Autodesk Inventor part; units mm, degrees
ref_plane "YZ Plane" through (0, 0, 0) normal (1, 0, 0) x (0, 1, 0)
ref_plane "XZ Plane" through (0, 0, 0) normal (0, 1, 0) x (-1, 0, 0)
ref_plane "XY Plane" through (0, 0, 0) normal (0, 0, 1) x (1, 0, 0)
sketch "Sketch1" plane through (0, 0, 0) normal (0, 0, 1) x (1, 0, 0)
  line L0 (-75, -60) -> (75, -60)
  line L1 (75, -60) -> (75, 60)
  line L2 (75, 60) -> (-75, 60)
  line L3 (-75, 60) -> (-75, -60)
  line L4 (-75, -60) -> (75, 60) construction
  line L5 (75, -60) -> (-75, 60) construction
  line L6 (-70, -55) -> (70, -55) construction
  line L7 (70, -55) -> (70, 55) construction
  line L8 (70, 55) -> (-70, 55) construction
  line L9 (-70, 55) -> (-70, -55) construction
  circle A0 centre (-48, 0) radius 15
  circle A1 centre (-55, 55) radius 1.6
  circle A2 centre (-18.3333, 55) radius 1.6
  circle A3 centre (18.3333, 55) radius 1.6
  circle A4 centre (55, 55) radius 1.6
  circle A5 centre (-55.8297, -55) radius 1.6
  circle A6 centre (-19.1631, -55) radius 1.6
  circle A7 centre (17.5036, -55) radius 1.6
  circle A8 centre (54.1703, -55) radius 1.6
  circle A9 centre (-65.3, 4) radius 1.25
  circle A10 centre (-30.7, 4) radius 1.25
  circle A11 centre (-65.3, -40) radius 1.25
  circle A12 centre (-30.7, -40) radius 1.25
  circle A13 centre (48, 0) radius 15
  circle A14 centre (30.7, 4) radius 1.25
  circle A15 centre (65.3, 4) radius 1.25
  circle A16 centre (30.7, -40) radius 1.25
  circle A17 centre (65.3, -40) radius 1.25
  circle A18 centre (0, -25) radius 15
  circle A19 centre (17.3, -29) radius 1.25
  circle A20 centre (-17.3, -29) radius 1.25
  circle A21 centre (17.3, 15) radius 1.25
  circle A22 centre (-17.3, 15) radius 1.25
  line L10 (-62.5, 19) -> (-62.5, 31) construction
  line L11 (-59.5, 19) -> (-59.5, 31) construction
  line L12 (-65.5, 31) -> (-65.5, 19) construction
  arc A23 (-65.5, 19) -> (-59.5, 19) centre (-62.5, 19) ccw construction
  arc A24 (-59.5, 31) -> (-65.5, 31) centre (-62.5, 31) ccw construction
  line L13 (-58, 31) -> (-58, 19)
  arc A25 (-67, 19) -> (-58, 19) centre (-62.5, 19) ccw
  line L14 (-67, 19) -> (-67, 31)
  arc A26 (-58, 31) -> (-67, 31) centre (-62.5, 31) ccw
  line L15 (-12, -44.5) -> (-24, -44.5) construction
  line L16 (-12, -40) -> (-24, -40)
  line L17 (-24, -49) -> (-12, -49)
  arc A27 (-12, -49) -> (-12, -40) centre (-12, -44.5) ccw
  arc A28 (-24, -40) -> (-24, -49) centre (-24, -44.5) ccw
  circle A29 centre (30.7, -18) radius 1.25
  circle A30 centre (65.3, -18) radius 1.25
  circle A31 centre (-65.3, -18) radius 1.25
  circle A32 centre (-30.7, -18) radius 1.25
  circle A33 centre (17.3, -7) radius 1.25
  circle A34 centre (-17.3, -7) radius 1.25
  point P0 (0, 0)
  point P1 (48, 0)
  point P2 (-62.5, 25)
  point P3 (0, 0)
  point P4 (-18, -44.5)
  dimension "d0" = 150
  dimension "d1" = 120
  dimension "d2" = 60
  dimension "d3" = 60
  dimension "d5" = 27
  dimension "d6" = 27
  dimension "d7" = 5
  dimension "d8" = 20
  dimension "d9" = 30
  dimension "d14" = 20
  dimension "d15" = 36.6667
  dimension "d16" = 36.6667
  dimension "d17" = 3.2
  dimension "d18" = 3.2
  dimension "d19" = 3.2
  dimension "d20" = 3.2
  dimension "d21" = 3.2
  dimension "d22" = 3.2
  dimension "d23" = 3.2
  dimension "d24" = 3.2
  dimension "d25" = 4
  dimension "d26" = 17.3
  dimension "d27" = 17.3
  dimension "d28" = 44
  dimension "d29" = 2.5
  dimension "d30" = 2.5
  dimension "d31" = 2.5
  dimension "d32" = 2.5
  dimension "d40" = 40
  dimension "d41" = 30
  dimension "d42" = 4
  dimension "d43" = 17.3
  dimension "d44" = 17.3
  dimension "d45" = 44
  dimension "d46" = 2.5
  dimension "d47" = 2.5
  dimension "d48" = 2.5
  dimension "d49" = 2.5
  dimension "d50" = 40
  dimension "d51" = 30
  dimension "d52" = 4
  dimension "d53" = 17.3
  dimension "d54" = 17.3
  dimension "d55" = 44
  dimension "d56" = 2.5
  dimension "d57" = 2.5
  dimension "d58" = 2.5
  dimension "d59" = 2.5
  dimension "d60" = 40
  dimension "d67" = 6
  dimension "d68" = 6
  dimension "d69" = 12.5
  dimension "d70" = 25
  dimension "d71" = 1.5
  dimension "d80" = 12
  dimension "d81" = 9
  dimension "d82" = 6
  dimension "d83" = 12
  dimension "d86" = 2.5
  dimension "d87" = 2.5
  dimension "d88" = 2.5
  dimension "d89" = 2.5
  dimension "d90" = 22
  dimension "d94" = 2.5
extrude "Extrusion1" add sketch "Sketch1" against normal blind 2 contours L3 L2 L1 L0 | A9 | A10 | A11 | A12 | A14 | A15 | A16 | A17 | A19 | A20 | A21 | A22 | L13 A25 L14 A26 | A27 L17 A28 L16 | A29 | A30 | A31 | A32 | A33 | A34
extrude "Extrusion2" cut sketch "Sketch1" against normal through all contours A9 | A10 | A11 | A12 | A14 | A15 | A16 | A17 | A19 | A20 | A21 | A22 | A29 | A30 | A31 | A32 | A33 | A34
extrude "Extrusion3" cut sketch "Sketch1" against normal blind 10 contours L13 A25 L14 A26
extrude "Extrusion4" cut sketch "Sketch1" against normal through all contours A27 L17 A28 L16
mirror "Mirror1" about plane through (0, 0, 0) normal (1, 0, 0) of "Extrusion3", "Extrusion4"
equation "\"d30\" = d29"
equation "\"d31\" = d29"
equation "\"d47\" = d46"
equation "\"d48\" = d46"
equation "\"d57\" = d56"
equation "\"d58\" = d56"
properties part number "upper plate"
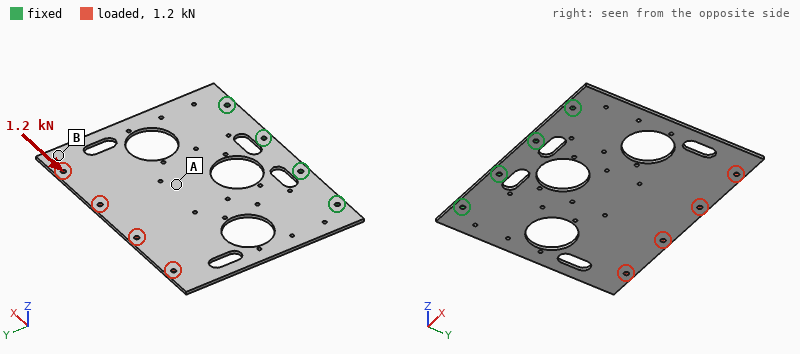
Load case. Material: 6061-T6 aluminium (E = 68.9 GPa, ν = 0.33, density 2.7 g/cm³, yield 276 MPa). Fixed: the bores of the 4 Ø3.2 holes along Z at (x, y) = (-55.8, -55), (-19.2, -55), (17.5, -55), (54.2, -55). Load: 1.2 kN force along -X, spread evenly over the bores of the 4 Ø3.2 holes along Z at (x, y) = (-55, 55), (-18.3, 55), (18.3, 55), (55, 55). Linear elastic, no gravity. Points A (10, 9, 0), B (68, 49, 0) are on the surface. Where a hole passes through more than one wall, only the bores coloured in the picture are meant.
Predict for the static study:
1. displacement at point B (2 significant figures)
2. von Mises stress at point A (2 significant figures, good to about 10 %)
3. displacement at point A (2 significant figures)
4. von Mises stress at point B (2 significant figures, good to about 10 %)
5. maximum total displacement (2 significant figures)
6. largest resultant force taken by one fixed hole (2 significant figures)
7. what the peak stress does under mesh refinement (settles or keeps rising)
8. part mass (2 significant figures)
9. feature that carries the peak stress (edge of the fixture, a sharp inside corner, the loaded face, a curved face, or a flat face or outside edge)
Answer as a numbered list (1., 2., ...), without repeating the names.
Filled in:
1. 72 µm
2. 18 MPa
3. 38 µm
4. 6.1 MPa
5. 79 µm
6. 1.2 kN
7. keeps rising
8. 81 g
9. edge of the fixture
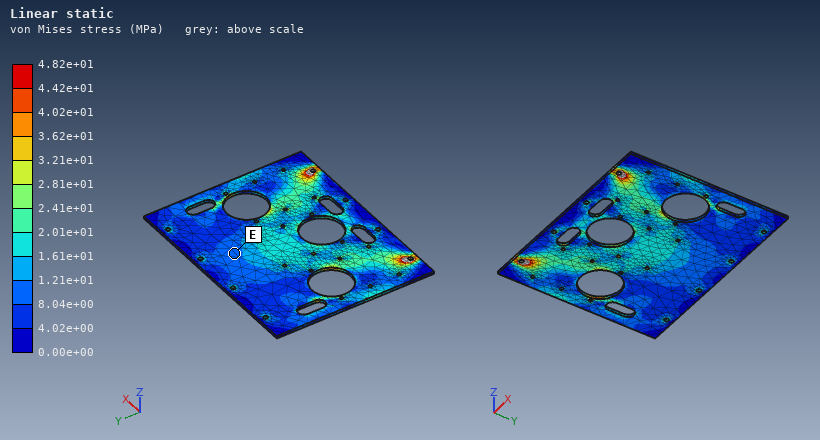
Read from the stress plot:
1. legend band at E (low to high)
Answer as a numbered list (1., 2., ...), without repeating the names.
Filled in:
1. 8.04e+00 to 1.21e+01 MPa
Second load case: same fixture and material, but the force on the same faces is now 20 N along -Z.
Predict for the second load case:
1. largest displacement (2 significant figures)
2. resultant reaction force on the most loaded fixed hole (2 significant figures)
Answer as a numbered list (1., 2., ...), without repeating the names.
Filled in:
1. 2.3 mm
2. 11 N
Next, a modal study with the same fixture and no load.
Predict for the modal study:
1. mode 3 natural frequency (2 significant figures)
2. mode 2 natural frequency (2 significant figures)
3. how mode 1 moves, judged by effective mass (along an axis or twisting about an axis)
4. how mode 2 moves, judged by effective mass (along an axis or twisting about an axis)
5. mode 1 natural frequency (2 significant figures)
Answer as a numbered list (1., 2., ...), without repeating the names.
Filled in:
1. 600 Hz
2. 240 Hz
3. along Z
4. twisting about Y
5. 100 Hz
